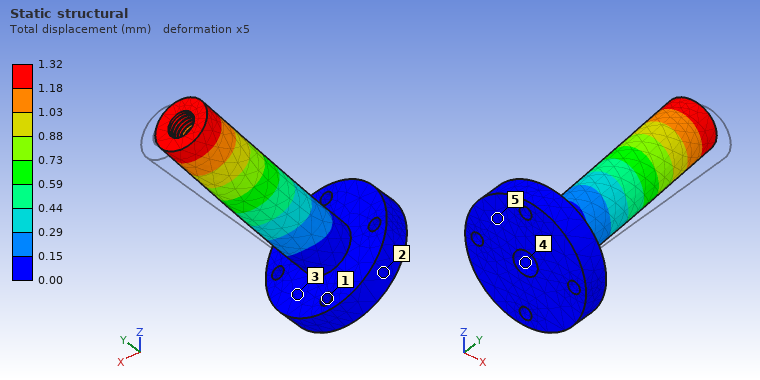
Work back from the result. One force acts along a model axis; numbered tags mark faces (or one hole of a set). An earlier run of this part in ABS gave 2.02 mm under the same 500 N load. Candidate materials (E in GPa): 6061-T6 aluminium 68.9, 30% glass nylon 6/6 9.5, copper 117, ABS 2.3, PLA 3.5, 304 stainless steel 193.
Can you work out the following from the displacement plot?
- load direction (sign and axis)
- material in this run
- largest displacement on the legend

-X
PLA
1.32 mm
